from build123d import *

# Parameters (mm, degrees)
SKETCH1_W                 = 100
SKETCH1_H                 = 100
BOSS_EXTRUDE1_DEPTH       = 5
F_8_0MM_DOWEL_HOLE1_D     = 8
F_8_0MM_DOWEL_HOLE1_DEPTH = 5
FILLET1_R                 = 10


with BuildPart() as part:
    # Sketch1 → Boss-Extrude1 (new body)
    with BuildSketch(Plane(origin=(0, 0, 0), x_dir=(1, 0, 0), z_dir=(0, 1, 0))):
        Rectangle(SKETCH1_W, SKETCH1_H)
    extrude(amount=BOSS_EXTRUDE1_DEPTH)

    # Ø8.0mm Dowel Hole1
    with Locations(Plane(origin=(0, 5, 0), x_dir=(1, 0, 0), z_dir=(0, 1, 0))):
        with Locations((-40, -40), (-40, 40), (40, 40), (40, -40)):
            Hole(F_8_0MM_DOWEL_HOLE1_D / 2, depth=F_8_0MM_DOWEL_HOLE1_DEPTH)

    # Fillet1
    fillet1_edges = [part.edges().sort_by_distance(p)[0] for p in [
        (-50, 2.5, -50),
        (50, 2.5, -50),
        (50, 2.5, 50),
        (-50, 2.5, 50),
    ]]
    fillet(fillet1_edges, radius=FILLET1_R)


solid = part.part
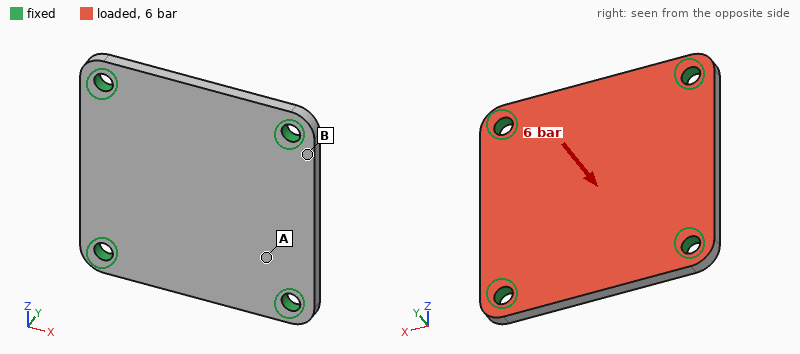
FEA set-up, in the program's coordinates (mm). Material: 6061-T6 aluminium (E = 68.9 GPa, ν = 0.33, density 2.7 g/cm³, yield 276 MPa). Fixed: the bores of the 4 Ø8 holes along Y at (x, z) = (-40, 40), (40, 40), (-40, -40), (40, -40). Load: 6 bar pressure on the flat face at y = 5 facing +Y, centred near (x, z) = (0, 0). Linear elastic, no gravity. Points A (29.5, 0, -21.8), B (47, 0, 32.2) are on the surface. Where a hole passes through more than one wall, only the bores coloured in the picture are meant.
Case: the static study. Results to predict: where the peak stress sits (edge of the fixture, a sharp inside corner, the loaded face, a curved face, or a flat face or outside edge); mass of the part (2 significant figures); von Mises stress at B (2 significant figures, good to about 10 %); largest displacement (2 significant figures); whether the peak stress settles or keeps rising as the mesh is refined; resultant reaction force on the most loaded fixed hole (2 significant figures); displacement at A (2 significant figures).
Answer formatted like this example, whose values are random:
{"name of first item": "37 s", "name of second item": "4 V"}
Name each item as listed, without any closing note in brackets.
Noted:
{"where the peak stress sits": "edge of the fixture", "mass of the part": "130 g", "von Mises stress at B": "54 MPa", "largest displacement": "0.19 mm", "whether the peak stress settles or keeps rising as the mesh is refined": "keeps rising", "resultant reaction force on the most loaded fixed hole": "1.5 kN", "displacement at A": "0.083 mm"}
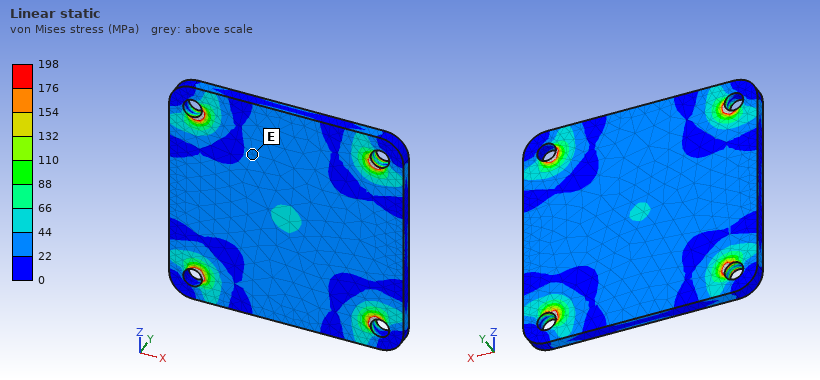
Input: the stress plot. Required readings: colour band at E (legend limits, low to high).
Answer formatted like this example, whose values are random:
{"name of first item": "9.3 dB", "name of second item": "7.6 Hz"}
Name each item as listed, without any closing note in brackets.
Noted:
{"colour band at E": "22 to 44 MPa"}
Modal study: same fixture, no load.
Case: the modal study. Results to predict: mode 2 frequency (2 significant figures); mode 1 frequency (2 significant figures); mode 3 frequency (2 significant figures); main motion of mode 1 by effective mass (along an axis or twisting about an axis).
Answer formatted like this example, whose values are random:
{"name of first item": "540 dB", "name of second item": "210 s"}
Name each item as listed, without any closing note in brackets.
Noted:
{"mode 2 frequency": "4800 Hz", "mode 1 frequency": "3000 Hz", "mode 3 frequency": "4800 Hz", "main motion of mode 1 by effective mass": "along Y"}
